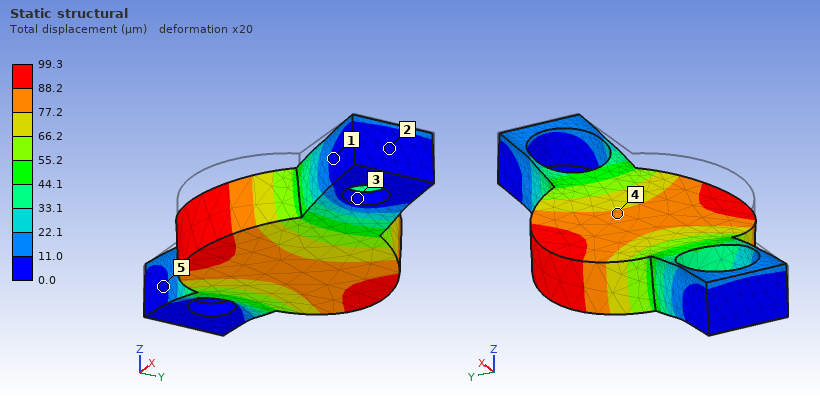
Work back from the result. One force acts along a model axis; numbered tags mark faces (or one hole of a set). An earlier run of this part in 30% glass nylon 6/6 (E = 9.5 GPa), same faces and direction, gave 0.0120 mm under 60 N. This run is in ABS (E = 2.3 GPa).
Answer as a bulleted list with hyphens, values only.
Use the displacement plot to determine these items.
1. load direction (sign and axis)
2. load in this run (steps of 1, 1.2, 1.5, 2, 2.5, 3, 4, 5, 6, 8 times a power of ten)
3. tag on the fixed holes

- -Z
- 120 N
- 3
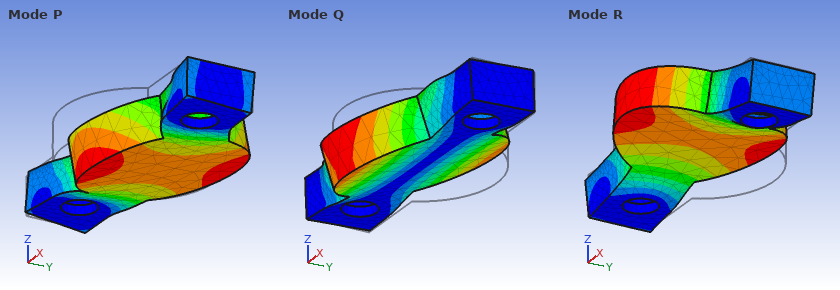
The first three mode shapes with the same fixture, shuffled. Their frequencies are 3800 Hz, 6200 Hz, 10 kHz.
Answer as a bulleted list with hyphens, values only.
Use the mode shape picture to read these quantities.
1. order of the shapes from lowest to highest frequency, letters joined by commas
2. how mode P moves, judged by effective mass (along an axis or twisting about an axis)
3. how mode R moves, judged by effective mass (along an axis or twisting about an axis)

- Q, R, P
- along Y
- along Z
